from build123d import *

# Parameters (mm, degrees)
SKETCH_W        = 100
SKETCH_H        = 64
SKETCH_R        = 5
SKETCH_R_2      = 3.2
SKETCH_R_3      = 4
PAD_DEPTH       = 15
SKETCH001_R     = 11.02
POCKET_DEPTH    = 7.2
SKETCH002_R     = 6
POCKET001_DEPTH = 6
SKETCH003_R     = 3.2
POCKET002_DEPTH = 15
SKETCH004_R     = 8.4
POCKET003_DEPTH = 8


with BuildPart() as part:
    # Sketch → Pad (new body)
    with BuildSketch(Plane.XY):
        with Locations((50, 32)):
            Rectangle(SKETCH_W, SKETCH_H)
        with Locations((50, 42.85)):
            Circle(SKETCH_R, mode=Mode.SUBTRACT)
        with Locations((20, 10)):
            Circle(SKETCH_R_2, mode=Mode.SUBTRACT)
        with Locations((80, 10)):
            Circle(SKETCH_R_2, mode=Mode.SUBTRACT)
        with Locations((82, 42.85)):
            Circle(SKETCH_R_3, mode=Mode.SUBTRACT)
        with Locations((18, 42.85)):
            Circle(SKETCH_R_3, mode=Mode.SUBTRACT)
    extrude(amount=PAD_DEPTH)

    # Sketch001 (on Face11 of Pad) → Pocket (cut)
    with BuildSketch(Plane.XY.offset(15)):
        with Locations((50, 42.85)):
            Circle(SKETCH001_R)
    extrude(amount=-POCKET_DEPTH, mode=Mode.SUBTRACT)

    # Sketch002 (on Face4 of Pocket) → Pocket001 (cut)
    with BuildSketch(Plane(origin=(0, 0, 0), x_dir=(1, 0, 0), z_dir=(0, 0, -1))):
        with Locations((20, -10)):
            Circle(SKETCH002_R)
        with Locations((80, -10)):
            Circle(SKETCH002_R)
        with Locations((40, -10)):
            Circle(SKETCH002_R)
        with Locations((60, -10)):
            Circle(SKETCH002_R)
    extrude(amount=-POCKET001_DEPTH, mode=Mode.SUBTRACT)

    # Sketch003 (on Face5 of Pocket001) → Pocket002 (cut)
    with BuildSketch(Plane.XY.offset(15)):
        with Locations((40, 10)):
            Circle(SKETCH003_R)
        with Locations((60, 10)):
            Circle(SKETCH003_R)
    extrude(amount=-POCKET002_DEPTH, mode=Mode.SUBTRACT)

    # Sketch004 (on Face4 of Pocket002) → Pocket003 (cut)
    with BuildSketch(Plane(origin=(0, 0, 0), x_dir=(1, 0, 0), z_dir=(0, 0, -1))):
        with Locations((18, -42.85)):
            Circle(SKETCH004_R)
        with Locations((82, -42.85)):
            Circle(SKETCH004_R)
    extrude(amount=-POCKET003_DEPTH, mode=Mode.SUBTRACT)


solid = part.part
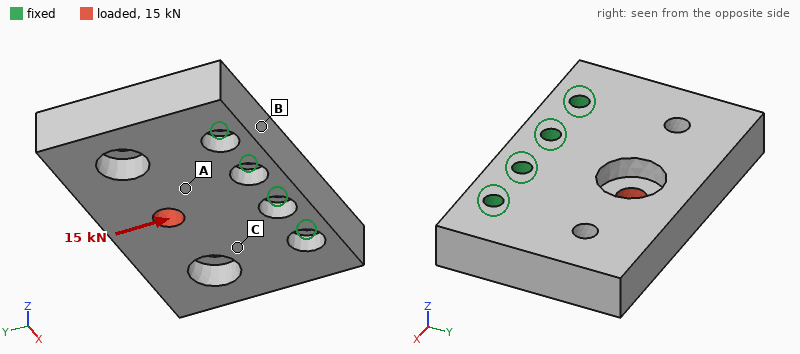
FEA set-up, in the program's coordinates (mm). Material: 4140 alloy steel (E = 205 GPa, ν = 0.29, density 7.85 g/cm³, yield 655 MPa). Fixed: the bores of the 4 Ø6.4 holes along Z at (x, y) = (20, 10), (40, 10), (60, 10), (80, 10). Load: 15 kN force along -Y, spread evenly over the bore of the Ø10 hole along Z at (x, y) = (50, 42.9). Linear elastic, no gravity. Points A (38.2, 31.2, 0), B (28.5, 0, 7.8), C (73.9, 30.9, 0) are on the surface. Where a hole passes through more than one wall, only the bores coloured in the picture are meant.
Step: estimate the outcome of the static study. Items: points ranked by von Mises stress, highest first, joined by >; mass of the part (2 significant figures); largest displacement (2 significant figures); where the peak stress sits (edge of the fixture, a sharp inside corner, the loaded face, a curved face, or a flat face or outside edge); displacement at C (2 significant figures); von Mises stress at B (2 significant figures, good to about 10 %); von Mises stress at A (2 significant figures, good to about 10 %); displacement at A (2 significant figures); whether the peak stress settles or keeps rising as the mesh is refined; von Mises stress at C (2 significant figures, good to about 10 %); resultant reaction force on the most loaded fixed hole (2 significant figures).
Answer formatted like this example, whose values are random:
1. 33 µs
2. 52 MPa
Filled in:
1. A > C > B
2. 660 g
3. 32 µm
4. edge of the fixture
5. 9.9 µm
6. 11 MPa
7. 38 MPa
8. 11 µm
9. keeps rising
10. 26 MPa
11. 4.6 kN
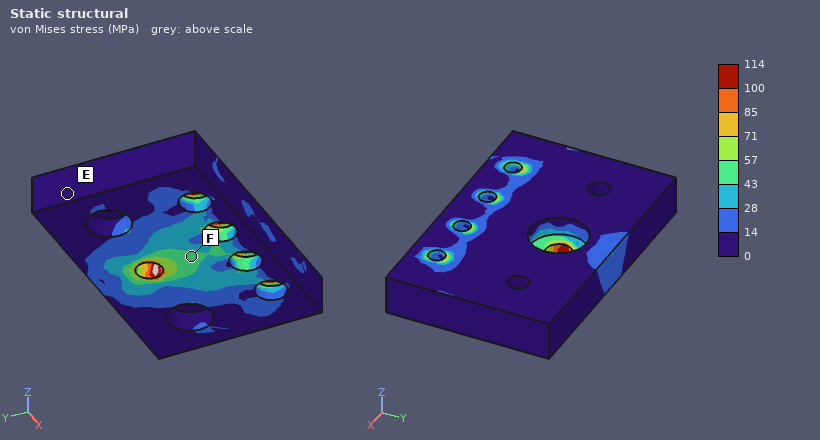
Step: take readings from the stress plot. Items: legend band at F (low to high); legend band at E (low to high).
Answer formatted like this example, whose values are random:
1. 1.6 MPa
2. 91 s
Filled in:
1. 43 to 57 MPa
2. 0 to 14 MPa
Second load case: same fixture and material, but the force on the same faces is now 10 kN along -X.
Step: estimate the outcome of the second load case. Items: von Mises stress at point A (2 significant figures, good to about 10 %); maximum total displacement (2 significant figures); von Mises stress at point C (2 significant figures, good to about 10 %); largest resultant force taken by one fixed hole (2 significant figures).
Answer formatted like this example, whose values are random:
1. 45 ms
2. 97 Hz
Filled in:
1. 29 MPa
2. 9.9 µm
3. 17 MPa
4. 5.4 kN
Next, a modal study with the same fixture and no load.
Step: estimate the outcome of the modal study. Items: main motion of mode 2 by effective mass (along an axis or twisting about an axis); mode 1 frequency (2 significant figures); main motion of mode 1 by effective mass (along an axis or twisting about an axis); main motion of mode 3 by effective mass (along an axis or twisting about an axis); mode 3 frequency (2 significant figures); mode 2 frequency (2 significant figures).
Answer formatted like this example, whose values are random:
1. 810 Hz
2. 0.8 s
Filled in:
1. twisting about Y
2. 3000 Hz
3. along Z
4. along X
5. 8600 Hz
6. 4500 Hz
